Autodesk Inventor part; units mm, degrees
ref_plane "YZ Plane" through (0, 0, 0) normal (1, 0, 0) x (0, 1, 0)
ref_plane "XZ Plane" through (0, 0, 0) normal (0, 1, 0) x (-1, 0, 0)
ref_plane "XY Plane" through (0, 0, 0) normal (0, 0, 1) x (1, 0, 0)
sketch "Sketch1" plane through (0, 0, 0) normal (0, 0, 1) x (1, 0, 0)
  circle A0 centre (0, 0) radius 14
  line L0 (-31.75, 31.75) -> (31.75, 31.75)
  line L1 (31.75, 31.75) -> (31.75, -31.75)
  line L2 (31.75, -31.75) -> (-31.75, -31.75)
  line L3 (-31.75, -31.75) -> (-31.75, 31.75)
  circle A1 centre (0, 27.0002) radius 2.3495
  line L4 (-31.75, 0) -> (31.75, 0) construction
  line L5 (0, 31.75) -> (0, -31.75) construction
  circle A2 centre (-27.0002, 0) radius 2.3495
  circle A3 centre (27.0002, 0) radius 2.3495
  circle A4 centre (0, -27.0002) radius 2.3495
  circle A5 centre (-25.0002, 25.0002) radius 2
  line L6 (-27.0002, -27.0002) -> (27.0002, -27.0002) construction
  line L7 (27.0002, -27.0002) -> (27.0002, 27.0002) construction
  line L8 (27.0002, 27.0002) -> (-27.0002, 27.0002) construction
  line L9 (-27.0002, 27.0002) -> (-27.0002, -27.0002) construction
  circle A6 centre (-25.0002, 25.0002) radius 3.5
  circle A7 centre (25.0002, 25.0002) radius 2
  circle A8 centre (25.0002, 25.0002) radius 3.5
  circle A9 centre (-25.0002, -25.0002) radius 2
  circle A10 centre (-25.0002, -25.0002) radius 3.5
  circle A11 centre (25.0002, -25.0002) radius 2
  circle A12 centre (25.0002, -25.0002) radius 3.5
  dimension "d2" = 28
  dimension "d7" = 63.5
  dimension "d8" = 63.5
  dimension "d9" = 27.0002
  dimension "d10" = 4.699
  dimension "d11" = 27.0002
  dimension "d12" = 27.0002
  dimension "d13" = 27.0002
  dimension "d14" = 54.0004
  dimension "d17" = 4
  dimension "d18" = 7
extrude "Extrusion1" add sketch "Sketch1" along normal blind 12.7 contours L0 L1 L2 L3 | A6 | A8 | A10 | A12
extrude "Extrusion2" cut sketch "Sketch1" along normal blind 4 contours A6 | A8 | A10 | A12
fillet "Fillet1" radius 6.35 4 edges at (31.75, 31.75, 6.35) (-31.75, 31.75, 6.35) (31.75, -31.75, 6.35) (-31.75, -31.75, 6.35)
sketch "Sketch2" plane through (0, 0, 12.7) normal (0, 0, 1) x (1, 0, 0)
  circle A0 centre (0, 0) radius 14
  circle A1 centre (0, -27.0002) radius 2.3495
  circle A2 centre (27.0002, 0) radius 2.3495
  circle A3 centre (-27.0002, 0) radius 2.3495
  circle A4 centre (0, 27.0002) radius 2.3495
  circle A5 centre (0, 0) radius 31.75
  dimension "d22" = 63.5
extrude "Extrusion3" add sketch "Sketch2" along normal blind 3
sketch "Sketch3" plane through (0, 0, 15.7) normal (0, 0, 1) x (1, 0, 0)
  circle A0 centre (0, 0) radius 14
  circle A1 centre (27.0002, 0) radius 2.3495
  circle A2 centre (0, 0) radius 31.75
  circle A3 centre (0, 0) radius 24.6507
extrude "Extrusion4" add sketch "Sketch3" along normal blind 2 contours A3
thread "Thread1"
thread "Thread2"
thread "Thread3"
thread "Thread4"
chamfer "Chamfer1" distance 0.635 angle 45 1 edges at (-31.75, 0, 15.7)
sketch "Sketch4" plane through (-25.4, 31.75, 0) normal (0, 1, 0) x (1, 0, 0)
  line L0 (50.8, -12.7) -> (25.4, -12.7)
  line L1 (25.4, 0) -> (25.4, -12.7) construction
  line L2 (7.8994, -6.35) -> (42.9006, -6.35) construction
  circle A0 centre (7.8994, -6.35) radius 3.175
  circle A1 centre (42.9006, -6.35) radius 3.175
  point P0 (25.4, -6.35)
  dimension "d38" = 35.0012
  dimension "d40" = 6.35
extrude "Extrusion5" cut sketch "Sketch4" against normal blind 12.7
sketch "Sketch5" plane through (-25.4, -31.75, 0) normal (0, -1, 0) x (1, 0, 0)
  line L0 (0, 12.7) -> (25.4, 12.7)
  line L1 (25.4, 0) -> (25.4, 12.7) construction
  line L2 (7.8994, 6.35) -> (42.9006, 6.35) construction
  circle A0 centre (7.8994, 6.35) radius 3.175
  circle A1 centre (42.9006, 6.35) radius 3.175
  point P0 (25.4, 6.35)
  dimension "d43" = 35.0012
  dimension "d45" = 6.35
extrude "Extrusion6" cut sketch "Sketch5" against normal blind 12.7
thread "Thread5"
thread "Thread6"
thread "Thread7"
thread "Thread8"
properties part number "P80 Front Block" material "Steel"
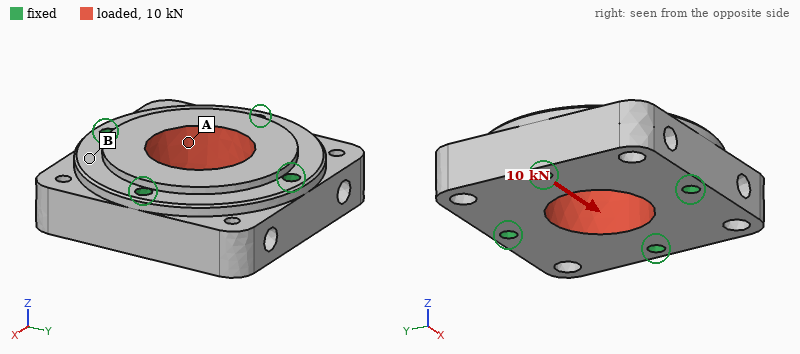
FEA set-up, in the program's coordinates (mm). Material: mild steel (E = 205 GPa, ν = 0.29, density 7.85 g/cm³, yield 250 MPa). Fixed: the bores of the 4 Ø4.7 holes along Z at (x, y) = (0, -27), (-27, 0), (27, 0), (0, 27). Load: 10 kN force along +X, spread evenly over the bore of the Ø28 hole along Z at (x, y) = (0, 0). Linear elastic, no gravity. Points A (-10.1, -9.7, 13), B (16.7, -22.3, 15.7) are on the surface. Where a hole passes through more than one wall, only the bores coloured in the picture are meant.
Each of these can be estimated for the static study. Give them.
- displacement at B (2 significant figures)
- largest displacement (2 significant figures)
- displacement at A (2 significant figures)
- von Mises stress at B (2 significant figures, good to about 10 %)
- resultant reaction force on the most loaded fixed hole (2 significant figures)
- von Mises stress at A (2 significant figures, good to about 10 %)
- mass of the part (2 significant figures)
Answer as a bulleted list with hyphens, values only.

- 0.72 µm
- 1.2 µm
- 1.1 µm
- 4.4 MPa
- 2.7 kN
- 9.7 MPa
- 390 g
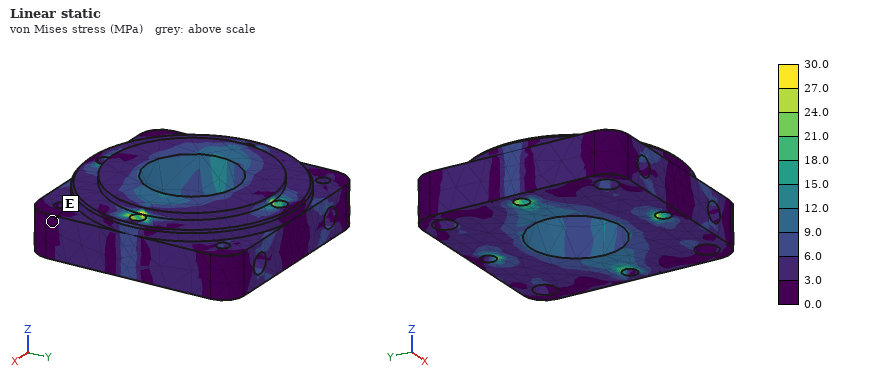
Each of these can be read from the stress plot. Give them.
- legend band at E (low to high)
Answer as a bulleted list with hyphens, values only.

- 0.0 to 3.0 MPa
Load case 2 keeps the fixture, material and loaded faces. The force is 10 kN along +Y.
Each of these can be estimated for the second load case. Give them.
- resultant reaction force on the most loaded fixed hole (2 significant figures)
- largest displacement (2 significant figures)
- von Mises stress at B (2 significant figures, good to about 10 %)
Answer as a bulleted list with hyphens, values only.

- 2.7 kN
- 1.1 µm
- 3.8 MPa
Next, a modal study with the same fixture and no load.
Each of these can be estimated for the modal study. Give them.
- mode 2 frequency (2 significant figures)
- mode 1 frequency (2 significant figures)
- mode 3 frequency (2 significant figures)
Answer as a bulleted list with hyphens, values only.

- 20 kHz
- 19 kHz
- 20 kHz
